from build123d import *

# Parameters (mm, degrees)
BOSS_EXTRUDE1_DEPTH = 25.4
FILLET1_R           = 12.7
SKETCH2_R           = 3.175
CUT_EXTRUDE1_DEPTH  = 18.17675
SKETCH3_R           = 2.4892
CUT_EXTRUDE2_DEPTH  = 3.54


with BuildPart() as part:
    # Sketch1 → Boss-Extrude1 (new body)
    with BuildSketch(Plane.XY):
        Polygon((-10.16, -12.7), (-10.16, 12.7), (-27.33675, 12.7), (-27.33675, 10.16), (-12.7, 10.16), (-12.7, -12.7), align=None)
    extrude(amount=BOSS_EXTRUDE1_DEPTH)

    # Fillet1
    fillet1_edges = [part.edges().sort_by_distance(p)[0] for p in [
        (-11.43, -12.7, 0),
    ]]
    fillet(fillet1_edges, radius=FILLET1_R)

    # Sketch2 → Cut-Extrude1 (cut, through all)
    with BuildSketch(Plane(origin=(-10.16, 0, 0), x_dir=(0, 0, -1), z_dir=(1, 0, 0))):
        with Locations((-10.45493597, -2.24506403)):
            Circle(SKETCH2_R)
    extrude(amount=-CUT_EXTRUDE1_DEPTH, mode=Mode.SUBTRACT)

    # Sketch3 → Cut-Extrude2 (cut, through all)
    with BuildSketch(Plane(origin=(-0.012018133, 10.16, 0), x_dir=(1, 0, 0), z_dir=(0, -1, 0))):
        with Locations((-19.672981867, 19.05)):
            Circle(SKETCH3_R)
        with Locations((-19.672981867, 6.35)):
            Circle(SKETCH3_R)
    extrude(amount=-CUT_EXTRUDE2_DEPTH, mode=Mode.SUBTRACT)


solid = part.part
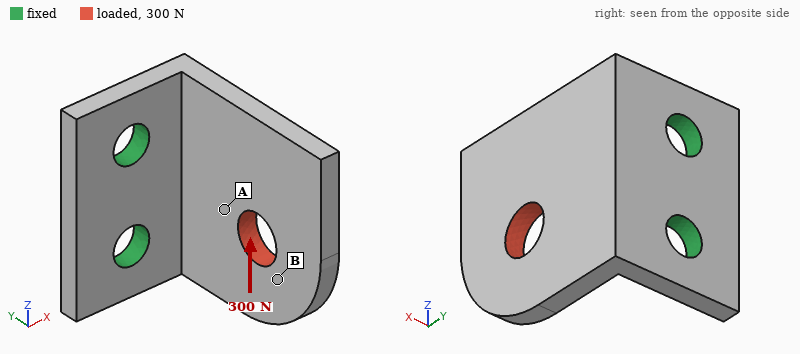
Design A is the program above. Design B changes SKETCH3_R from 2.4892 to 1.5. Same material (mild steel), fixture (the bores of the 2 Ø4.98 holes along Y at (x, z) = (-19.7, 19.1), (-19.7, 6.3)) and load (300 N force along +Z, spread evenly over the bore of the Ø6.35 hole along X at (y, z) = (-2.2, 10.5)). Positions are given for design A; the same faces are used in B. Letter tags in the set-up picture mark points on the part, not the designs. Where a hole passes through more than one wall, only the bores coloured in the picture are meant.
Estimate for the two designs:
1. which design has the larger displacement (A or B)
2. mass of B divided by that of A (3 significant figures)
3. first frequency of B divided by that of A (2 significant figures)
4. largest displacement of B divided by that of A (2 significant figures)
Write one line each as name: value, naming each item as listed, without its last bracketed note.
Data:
which design has the larger displacement: B
mass of B divided by that of A: 1.03
first frequency of B divided by that of A: 0.94
largest displacement of B divided by that of A: 1.4
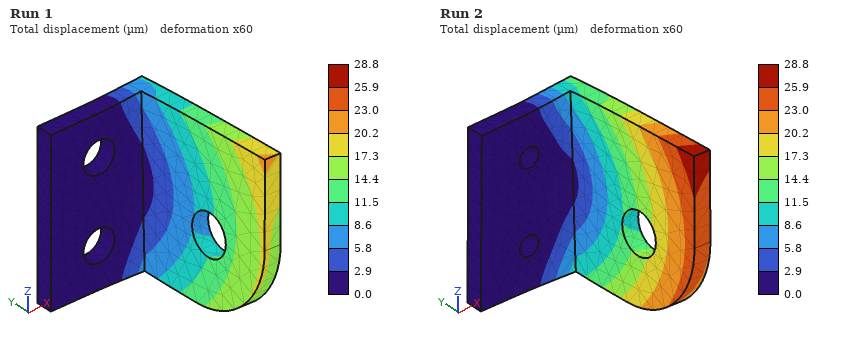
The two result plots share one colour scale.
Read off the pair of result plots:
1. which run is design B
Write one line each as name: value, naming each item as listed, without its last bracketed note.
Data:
which run is design B: Run 2
